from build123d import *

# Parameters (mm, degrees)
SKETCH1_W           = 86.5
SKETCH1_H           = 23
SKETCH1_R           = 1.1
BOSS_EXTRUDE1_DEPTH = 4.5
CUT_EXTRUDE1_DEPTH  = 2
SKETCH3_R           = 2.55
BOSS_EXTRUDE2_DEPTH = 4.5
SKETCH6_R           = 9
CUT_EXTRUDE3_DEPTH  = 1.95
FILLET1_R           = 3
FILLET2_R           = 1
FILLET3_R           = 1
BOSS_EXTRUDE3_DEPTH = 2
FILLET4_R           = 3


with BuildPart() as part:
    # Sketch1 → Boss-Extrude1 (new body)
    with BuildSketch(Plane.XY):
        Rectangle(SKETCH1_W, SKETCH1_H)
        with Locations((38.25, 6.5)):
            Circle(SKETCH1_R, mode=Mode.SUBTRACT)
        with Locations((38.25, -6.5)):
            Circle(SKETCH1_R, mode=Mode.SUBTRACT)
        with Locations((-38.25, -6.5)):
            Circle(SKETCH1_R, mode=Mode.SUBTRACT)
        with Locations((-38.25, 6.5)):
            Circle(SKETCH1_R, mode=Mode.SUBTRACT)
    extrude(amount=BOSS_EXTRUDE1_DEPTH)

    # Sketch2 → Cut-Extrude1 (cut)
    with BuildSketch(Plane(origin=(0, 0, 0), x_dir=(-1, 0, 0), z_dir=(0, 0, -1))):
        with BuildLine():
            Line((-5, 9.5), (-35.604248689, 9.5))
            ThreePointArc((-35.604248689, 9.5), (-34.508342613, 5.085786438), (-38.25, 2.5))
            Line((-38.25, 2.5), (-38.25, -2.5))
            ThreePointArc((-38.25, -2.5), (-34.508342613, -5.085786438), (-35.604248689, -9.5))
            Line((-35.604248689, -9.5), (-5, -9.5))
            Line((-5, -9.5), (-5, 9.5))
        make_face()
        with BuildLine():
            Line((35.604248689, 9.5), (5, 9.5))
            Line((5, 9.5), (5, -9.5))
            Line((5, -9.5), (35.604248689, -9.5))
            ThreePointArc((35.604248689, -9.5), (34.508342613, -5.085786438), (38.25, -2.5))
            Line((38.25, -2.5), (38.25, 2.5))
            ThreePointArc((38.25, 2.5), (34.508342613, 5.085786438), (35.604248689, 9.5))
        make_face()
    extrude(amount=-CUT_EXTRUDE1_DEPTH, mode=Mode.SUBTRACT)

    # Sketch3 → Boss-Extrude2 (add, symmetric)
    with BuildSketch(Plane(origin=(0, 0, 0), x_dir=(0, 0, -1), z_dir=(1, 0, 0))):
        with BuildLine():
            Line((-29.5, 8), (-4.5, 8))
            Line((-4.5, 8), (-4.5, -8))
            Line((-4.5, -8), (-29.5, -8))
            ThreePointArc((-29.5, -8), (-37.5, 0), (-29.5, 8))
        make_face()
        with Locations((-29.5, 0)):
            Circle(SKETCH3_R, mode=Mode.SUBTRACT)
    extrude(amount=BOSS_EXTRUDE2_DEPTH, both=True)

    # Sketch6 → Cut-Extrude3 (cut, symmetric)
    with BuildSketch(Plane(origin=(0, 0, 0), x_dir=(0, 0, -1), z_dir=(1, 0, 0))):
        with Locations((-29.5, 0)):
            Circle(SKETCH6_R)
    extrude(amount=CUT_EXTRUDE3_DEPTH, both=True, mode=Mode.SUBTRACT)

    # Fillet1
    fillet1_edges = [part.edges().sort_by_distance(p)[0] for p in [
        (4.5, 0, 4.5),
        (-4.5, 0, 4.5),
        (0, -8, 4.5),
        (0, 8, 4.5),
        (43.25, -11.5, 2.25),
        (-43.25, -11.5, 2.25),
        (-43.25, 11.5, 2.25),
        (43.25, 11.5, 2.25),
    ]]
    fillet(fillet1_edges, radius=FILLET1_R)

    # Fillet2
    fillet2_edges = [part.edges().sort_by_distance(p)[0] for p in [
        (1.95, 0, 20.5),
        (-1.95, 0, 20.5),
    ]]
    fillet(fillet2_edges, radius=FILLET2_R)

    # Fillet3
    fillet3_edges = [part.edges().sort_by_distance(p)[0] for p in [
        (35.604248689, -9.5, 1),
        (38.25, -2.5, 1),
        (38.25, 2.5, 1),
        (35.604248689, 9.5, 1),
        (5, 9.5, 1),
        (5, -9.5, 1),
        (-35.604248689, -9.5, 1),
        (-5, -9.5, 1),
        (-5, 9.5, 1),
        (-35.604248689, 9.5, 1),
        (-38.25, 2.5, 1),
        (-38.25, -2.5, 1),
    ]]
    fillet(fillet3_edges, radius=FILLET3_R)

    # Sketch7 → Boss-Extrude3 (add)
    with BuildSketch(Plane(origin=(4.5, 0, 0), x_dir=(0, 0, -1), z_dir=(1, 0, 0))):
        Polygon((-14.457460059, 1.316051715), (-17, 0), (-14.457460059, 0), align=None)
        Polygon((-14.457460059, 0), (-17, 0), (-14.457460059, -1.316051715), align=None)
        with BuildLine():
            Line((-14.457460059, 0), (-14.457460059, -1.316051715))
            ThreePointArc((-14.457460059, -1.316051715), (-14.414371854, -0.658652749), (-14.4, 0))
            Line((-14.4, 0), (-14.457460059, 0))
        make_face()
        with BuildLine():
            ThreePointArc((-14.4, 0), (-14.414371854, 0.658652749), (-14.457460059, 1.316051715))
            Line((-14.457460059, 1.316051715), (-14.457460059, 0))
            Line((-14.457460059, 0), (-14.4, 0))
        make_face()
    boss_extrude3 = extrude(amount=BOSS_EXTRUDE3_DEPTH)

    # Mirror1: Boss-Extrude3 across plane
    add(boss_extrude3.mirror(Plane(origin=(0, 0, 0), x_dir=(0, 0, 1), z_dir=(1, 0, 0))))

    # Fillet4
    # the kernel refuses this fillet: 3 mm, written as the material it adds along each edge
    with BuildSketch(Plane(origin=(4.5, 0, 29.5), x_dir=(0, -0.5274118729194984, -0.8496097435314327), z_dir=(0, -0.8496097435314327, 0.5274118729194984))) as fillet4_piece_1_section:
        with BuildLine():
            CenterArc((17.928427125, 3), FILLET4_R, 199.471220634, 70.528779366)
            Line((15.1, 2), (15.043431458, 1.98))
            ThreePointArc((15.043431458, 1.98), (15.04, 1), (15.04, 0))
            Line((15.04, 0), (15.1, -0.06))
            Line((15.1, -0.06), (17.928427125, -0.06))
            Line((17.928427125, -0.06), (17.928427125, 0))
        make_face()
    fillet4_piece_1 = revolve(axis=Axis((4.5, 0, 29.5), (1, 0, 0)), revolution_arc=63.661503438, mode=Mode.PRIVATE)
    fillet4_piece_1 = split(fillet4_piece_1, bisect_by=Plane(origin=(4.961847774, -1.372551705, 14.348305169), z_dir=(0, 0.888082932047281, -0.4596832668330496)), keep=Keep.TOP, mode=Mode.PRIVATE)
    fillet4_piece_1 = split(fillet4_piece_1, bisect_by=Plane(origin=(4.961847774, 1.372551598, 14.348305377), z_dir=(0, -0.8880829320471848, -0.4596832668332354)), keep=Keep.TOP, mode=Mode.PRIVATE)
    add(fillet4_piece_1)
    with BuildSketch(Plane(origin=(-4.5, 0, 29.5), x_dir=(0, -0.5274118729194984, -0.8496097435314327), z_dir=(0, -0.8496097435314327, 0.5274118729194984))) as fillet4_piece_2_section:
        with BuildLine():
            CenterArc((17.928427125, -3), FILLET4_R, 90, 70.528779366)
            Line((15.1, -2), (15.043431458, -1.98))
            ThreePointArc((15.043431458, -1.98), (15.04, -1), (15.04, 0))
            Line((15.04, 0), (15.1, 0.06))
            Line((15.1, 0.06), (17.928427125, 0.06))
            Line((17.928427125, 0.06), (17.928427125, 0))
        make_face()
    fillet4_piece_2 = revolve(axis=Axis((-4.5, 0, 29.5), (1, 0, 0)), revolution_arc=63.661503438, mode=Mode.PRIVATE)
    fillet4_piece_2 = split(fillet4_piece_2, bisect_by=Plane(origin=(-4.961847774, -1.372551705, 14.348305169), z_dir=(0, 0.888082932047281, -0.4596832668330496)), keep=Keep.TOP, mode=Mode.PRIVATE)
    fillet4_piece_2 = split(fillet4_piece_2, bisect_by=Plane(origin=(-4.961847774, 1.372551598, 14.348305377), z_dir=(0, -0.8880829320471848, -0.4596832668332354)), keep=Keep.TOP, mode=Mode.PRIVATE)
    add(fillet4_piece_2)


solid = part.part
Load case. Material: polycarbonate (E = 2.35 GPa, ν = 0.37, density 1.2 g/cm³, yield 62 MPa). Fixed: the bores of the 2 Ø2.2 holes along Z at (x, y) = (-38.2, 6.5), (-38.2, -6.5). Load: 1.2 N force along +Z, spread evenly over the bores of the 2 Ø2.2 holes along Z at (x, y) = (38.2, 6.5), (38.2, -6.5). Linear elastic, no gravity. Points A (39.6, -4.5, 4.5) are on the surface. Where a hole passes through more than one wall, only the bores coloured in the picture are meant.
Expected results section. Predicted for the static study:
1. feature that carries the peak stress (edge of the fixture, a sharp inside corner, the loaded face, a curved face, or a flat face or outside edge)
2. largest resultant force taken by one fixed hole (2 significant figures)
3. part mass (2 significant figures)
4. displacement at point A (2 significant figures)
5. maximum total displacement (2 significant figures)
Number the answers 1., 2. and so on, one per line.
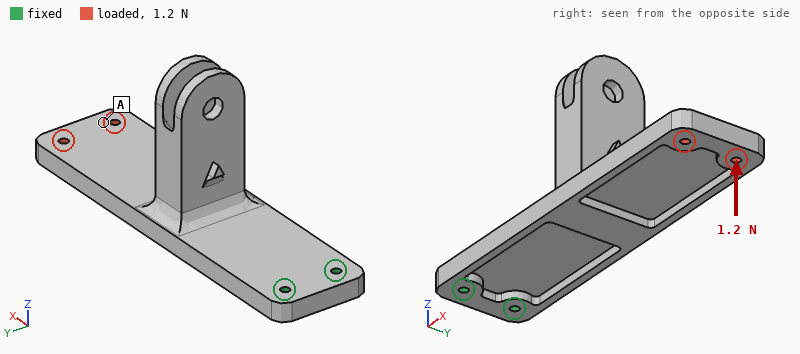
1. a curved face
2. 1.7 N
3. 12 g
4. 1.00 mm
5. 1.1 mm
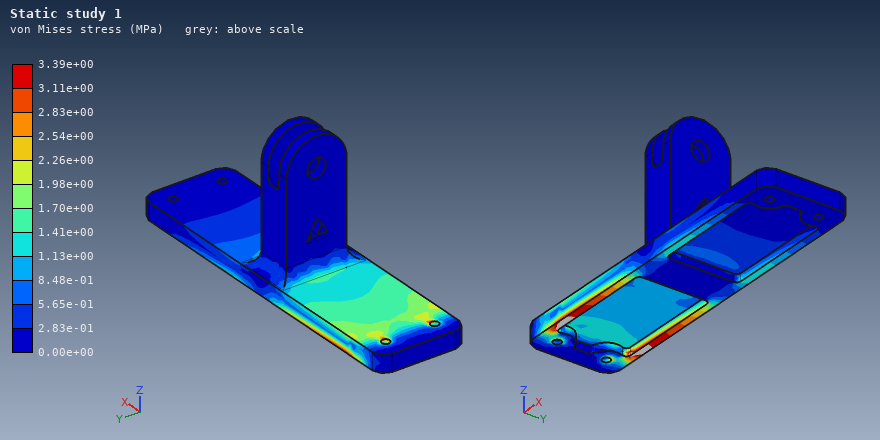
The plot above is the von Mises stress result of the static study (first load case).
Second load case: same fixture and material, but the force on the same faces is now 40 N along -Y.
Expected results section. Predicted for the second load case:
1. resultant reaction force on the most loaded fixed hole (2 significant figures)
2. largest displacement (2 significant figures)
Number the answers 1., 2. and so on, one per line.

1. 210 N
2. 1.0 mm
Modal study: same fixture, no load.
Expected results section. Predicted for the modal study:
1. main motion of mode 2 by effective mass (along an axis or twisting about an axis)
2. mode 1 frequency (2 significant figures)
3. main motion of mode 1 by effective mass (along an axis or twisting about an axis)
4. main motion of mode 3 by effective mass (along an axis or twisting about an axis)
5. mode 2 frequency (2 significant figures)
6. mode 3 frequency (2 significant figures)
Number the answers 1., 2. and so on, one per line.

1. along Y
2. 100 Hz
3. along Z
4. along Z
5. 330 Hz
6. 570 Hz
